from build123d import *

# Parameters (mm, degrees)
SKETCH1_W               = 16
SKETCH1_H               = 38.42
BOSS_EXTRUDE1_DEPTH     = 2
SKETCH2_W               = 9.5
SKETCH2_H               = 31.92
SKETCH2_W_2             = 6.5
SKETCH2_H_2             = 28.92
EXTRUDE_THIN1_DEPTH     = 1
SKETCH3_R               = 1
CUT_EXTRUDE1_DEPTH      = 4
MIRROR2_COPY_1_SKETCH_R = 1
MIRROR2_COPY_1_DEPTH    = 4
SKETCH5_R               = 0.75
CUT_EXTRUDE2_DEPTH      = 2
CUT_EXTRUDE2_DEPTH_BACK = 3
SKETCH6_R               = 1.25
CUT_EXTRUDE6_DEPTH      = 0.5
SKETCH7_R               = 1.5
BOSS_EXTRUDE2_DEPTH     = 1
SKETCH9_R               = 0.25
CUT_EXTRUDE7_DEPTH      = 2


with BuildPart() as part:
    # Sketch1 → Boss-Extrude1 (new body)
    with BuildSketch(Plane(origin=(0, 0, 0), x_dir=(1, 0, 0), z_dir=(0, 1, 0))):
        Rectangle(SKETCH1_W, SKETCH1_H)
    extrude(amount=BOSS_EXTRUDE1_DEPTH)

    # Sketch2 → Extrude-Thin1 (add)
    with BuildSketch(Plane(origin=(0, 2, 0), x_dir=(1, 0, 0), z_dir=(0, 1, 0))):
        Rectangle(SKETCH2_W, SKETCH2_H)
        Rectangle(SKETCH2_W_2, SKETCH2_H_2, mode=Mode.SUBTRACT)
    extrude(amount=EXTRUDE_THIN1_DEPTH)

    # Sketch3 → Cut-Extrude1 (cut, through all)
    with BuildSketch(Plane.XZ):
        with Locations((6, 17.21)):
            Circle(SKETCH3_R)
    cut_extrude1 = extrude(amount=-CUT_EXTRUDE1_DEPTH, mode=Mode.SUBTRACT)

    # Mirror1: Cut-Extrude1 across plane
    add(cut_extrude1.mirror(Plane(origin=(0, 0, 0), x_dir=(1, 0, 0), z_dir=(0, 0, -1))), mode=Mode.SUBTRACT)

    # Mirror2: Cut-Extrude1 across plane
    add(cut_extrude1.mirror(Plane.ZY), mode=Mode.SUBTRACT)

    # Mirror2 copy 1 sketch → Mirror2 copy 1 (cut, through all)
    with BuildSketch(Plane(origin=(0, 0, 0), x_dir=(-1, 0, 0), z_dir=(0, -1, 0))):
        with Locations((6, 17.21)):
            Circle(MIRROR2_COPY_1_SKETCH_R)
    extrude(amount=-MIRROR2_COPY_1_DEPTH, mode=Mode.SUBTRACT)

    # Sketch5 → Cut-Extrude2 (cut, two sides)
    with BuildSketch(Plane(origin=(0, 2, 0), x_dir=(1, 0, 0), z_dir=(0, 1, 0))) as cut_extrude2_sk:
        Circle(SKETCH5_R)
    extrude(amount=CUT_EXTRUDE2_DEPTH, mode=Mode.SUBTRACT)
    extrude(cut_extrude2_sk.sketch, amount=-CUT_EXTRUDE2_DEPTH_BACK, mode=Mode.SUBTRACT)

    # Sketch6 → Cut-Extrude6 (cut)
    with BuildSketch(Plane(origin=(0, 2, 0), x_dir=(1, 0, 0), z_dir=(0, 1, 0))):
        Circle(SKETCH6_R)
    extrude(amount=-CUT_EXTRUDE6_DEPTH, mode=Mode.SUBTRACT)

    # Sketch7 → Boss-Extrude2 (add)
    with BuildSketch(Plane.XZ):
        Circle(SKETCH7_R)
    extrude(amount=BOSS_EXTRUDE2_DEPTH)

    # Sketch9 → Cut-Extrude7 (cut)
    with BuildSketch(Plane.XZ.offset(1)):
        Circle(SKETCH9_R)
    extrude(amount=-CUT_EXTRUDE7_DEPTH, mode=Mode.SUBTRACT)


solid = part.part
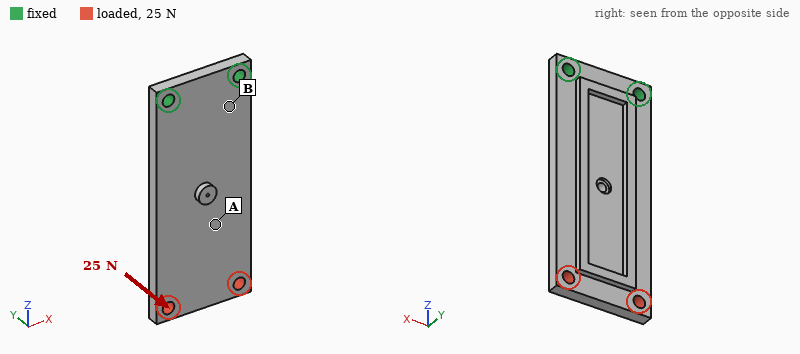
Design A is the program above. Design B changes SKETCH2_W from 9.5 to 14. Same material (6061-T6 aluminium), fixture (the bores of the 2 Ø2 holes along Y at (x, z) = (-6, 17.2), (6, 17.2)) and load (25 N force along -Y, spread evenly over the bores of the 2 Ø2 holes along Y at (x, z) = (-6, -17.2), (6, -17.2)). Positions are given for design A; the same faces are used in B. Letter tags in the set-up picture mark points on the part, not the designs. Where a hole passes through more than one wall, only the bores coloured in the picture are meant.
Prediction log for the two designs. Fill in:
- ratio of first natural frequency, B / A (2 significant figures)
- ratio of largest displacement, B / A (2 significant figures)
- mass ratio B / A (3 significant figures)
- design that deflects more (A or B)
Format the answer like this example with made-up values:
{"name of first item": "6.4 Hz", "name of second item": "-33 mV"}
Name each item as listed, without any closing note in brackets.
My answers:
{"ratio of first natural frequency, B / A": "1.1", "ratio of largest displacement, B / A": "0.74", "mass ratio B / A": "1.11", "design that deflects more": "A"}
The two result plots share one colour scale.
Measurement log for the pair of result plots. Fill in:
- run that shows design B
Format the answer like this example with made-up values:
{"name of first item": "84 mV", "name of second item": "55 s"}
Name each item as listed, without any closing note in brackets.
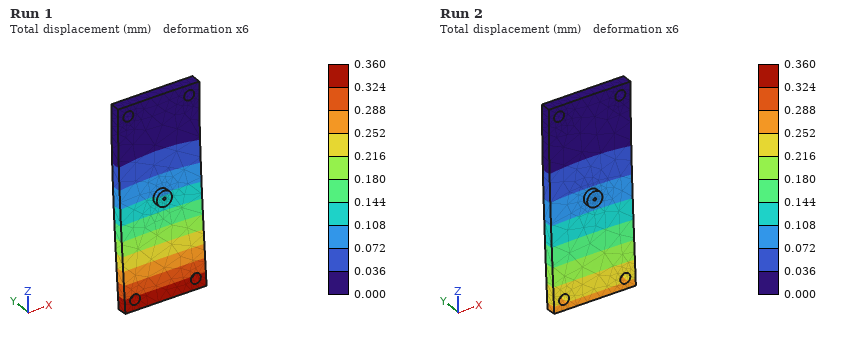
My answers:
{"run that shows design B": "Run 2"}
